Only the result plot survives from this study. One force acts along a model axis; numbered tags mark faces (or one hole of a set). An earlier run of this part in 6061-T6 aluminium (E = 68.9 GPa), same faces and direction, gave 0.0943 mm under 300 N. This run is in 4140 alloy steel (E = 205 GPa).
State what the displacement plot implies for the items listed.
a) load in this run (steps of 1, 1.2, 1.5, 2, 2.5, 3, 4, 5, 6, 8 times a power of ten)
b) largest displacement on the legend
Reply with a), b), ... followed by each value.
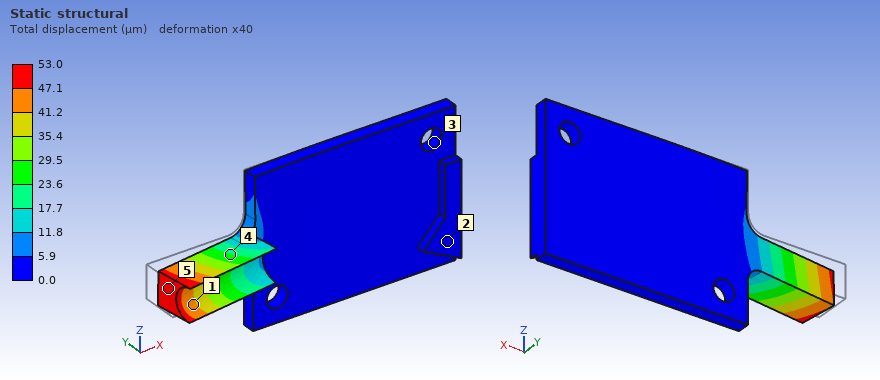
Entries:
a) 500 N
b) 53.0 µm
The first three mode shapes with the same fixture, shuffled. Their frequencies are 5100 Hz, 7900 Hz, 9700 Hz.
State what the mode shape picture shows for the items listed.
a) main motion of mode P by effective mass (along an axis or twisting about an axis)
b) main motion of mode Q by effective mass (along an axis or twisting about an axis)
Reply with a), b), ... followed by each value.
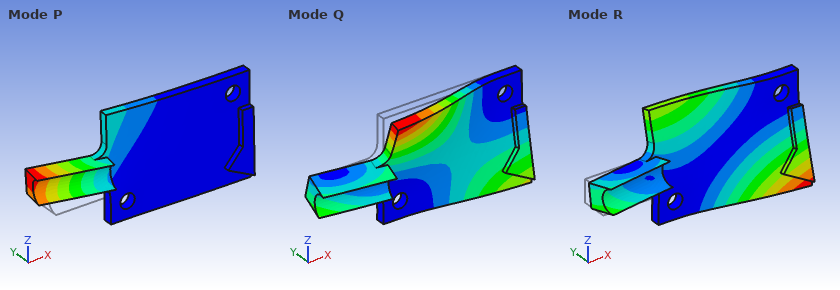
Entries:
a) along Y
b) along Y
